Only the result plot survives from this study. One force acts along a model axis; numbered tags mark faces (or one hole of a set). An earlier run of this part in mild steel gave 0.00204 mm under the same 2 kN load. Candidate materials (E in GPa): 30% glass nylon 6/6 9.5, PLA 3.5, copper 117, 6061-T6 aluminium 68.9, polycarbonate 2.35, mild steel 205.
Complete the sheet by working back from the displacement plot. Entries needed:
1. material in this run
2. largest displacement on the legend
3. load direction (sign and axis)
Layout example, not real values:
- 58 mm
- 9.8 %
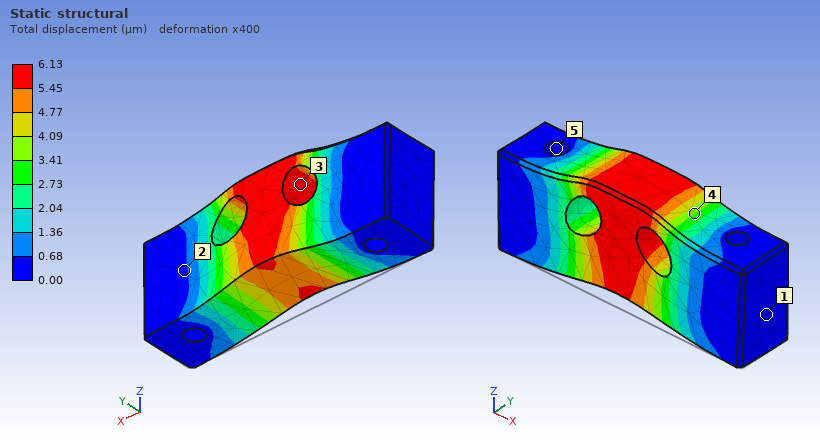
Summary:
- 6061-T6 aluminium
- 6.13 µm
- +Z
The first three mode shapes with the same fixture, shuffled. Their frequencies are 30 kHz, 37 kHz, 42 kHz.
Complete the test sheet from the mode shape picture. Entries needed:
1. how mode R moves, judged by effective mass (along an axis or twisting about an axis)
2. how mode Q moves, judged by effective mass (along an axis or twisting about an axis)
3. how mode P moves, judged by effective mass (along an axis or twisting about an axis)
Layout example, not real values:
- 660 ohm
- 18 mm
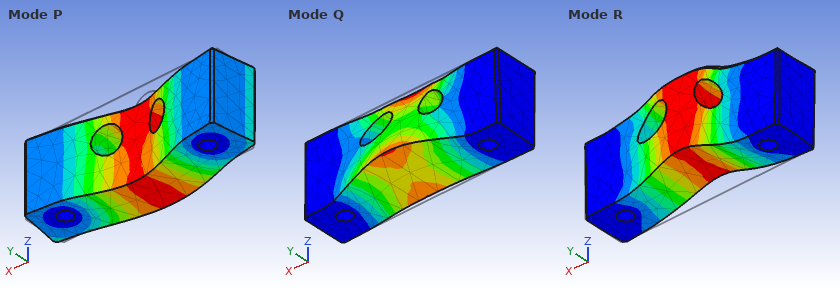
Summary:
- along Z
- twisting about X
- along Y
